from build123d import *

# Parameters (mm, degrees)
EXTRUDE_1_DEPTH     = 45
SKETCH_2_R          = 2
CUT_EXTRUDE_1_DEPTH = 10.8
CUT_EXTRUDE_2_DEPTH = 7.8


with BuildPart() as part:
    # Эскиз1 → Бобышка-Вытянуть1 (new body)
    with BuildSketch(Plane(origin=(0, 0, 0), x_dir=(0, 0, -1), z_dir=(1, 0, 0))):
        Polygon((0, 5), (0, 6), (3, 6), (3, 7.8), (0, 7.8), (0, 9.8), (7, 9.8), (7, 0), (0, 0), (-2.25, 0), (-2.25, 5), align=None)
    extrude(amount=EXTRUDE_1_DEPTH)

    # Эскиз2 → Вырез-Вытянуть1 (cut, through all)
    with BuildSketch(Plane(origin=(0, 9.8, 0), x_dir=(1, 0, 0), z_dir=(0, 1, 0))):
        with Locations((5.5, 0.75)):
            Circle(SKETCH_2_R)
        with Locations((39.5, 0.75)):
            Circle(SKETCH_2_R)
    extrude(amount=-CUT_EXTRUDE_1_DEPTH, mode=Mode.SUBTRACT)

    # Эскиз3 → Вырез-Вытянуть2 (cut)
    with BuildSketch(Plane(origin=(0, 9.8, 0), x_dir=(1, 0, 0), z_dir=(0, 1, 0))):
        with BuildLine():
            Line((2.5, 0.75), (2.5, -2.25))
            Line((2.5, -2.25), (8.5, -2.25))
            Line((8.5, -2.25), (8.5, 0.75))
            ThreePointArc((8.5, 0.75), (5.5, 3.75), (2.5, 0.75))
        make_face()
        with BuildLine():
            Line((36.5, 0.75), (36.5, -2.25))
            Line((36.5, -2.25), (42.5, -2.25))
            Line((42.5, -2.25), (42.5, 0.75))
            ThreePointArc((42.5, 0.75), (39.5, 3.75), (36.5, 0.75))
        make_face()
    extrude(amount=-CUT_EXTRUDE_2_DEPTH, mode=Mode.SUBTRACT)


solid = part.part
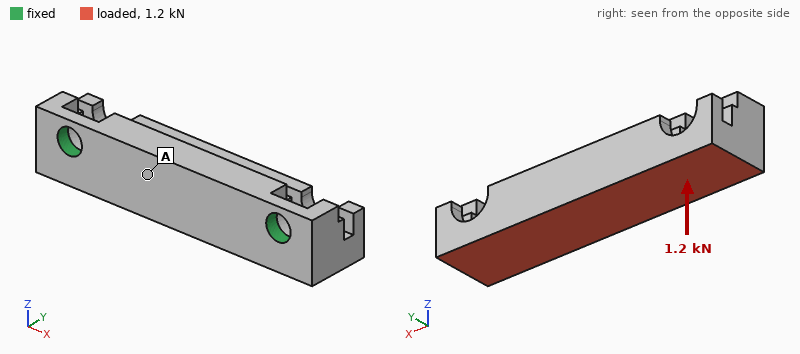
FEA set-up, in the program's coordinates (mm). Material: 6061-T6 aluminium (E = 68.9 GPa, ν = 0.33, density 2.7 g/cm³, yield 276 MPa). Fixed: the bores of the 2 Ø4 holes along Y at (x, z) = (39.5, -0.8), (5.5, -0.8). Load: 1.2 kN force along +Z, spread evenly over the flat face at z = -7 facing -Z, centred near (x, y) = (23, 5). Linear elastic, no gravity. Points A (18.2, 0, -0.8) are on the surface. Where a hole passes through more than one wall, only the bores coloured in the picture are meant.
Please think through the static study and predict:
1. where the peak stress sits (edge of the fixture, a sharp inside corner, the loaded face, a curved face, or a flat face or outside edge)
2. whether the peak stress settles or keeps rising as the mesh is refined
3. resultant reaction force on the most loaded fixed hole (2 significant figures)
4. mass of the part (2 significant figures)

edge of the fixture
keeps rising
610 N
8.1 g
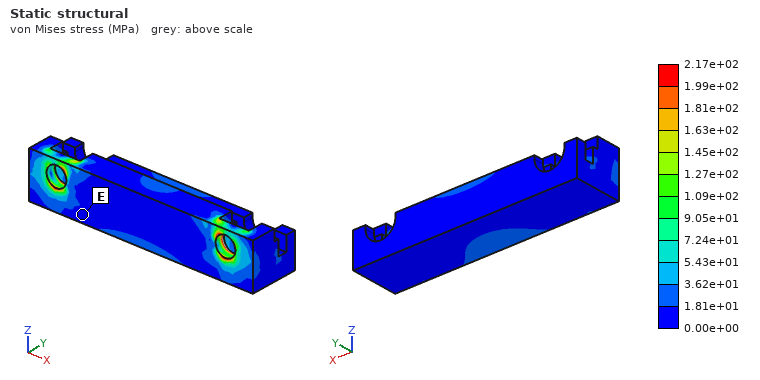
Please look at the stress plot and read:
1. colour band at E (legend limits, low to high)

0.00e+00 to 1.81e+01 MPa
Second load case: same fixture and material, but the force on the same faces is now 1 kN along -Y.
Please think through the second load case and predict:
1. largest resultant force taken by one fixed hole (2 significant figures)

540 N
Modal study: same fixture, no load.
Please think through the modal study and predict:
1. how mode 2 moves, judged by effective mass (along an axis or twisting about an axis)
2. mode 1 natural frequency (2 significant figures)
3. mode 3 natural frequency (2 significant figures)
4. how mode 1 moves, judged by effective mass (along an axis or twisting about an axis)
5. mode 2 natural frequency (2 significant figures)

along Y
12 kHz
23 kHz
along Z
21 kHz
